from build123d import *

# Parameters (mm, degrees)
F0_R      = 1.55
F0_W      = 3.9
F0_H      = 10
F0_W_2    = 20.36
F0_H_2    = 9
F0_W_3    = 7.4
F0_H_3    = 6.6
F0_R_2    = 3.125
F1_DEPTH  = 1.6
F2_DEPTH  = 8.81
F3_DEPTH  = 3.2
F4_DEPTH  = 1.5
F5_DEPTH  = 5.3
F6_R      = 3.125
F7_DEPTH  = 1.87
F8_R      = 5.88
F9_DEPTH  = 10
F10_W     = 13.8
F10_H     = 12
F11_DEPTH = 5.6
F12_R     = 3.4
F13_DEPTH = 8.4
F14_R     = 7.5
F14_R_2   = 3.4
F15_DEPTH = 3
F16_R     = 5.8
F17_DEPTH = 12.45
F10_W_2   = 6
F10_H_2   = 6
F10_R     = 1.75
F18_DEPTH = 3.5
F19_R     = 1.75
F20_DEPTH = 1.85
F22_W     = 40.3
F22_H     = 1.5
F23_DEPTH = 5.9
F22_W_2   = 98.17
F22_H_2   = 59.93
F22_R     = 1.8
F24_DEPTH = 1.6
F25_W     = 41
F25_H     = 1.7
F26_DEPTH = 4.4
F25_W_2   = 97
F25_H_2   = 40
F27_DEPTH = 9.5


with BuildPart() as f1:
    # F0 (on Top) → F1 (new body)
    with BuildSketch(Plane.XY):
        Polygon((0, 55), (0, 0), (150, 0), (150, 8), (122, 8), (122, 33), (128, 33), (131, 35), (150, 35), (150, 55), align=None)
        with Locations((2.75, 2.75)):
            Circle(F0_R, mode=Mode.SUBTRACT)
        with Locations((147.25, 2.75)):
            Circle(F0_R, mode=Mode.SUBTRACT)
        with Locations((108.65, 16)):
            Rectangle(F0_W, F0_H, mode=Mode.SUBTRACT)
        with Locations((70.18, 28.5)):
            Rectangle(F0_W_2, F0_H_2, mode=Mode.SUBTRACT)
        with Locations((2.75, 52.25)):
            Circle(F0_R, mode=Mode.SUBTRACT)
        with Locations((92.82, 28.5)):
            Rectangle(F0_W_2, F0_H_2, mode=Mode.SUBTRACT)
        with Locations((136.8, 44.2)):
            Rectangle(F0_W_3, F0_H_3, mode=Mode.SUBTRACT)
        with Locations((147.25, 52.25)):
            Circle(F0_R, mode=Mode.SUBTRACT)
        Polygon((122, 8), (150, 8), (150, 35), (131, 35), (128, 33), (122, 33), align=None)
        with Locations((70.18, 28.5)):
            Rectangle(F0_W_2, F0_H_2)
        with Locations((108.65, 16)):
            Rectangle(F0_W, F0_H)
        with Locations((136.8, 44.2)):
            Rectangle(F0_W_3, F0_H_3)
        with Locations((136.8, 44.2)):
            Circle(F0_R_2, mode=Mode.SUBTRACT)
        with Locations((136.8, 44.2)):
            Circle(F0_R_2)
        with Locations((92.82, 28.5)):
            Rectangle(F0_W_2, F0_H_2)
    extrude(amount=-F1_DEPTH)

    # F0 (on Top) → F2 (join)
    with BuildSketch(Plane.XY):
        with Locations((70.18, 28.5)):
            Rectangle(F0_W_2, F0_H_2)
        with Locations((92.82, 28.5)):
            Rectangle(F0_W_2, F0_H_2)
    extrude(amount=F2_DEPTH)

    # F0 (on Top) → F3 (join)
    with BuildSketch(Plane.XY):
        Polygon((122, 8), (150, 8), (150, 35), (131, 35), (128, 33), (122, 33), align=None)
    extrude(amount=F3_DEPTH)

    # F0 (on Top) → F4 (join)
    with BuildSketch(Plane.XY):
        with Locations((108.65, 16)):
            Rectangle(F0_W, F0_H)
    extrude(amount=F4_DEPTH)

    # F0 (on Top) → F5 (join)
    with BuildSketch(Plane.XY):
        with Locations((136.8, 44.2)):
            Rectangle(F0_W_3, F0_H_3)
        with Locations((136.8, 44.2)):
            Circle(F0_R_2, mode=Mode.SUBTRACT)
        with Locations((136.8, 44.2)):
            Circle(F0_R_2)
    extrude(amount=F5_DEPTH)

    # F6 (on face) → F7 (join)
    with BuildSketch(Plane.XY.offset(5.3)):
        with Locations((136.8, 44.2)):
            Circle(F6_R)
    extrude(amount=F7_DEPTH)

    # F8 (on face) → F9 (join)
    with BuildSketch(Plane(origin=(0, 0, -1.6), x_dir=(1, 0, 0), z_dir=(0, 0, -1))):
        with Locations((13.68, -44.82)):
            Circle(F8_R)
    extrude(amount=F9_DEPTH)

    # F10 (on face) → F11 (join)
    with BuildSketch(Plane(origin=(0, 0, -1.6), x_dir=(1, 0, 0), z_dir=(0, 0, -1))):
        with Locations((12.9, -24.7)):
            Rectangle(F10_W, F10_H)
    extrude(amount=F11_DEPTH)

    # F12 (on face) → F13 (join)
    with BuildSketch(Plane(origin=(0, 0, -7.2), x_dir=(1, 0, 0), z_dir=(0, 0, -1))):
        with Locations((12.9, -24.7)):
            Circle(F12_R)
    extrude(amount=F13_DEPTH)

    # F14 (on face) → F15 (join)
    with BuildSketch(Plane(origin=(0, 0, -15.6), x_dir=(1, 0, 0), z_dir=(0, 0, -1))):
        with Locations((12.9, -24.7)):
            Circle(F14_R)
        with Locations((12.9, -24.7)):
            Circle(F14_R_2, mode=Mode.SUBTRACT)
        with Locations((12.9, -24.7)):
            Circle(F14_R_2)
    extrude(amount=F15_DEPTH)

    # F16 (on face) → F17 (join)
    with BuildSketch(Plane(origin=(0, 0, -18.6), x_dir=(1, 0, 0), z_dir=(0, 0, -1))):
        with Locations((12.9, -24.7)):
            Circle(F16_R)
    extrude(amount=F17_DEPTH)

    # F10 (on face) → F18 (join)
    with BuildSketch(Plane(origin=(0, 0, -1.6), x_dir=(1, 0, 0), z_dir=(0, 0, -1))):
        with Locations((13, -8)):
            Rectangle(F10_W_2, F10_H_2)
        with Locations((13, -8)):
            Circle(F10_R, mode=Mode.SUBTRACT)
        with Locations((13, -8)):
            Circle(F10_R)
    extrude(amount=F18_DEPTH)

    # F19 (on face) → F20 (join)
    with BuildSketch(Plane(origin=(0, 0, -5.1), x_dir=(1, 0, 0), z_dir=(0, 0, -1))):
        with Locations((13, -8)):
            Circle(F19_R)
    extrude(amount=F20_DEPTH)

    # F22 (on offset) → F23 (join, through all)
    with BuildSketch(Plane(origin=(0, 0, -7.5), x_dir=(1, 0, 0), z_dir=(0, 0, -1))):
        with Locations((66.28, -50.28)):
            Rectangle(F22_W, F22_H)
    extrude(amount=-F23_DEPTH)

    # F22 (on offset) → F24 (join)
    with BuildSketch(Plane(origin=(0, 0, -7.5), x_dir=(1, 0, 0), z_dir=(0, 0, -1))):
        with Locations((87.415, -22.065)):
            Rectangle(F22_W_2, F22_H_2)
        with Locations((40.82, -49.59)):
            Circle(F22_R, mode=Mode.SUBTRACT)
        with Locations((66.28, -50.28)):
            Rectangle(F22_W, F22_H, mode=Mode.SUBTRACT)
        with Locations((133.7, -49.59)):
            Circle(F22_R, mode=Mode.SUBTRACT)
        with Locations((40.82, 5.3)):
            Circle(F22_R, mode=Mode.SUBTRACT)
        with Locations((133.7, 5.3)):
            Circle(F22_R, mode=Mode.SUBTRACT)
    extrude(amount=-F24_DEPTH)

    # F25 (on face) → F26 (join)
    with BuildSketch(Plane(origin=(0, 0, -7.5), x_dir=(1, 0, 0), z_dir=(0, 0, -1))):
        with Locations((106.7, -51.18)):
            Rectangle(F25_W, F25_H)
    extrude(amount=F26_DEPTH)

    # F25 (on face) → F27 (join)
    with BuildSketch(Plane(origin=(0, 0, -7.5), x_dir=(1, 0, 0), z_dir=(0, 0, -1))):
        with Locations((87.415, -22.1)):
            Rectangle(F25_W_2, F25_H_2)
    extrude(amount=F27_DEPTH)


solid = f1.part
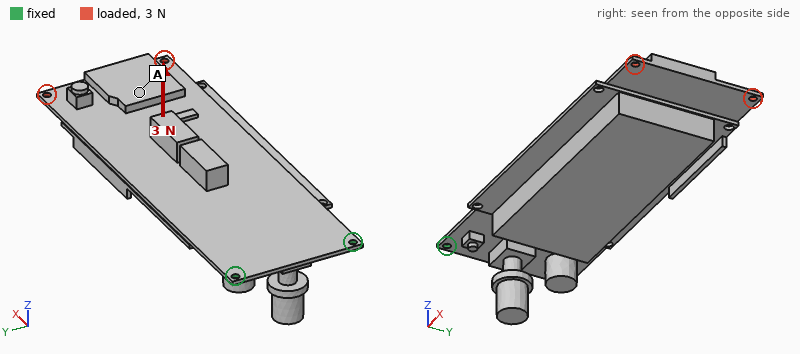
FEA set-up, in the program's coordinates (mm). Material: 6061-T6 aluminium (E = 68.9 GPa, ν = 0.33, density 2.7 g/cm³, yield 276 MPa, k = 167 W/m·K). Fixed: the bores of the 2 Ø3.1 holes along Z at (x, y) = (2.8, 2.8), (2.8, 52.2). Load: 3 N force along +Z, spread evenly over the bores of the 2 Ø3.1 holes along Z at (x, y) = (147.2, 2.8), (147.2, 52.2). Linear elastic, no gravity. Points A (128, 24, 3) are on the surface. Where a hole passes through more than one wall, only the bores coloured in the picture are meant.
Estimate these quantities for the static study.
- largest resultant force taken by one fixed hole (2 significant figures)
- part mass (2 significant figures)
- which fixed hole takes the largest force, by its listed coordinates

2.3 N
190 g
(2.8, 2.8)
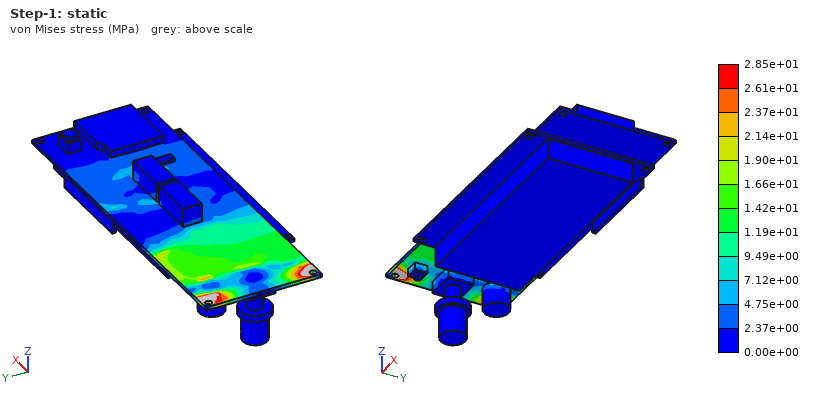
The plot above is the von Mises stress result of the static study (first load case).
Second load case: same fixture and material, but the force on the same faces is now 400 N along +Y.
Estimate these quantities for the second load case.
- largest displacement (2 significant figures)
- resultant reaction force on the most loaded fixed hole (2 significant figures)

0.37 mm
1.2 kN
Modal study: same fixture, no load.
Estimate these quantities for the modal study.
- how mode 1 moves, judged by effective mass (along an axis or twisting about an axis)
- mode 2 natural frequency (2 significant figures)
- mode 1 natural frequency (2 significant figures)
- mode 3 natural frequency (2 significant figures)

along Z
120 Hz
27 Hz
220 Hz
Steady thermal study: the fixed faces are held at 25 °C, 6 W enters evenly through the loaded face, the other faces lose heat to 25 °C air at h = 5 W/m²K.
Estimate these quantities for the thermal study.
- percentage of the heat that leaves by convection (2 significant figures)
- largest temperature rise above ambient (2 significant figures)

48 %
48 K
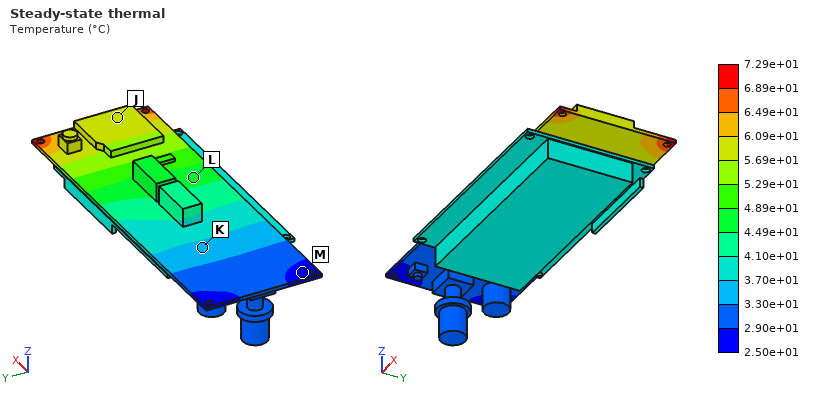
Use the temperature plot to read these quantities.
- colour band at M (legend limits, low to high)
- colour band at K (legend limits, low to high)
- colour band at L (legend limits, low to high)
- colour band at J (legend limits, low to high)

2.50e+01 to 2.90e+01 °C
3.30e+01 to 3.70e+01 °C
4.49e+01 to 4.89e+01 °C
5.69e+01 to 6.09e+01 °C
